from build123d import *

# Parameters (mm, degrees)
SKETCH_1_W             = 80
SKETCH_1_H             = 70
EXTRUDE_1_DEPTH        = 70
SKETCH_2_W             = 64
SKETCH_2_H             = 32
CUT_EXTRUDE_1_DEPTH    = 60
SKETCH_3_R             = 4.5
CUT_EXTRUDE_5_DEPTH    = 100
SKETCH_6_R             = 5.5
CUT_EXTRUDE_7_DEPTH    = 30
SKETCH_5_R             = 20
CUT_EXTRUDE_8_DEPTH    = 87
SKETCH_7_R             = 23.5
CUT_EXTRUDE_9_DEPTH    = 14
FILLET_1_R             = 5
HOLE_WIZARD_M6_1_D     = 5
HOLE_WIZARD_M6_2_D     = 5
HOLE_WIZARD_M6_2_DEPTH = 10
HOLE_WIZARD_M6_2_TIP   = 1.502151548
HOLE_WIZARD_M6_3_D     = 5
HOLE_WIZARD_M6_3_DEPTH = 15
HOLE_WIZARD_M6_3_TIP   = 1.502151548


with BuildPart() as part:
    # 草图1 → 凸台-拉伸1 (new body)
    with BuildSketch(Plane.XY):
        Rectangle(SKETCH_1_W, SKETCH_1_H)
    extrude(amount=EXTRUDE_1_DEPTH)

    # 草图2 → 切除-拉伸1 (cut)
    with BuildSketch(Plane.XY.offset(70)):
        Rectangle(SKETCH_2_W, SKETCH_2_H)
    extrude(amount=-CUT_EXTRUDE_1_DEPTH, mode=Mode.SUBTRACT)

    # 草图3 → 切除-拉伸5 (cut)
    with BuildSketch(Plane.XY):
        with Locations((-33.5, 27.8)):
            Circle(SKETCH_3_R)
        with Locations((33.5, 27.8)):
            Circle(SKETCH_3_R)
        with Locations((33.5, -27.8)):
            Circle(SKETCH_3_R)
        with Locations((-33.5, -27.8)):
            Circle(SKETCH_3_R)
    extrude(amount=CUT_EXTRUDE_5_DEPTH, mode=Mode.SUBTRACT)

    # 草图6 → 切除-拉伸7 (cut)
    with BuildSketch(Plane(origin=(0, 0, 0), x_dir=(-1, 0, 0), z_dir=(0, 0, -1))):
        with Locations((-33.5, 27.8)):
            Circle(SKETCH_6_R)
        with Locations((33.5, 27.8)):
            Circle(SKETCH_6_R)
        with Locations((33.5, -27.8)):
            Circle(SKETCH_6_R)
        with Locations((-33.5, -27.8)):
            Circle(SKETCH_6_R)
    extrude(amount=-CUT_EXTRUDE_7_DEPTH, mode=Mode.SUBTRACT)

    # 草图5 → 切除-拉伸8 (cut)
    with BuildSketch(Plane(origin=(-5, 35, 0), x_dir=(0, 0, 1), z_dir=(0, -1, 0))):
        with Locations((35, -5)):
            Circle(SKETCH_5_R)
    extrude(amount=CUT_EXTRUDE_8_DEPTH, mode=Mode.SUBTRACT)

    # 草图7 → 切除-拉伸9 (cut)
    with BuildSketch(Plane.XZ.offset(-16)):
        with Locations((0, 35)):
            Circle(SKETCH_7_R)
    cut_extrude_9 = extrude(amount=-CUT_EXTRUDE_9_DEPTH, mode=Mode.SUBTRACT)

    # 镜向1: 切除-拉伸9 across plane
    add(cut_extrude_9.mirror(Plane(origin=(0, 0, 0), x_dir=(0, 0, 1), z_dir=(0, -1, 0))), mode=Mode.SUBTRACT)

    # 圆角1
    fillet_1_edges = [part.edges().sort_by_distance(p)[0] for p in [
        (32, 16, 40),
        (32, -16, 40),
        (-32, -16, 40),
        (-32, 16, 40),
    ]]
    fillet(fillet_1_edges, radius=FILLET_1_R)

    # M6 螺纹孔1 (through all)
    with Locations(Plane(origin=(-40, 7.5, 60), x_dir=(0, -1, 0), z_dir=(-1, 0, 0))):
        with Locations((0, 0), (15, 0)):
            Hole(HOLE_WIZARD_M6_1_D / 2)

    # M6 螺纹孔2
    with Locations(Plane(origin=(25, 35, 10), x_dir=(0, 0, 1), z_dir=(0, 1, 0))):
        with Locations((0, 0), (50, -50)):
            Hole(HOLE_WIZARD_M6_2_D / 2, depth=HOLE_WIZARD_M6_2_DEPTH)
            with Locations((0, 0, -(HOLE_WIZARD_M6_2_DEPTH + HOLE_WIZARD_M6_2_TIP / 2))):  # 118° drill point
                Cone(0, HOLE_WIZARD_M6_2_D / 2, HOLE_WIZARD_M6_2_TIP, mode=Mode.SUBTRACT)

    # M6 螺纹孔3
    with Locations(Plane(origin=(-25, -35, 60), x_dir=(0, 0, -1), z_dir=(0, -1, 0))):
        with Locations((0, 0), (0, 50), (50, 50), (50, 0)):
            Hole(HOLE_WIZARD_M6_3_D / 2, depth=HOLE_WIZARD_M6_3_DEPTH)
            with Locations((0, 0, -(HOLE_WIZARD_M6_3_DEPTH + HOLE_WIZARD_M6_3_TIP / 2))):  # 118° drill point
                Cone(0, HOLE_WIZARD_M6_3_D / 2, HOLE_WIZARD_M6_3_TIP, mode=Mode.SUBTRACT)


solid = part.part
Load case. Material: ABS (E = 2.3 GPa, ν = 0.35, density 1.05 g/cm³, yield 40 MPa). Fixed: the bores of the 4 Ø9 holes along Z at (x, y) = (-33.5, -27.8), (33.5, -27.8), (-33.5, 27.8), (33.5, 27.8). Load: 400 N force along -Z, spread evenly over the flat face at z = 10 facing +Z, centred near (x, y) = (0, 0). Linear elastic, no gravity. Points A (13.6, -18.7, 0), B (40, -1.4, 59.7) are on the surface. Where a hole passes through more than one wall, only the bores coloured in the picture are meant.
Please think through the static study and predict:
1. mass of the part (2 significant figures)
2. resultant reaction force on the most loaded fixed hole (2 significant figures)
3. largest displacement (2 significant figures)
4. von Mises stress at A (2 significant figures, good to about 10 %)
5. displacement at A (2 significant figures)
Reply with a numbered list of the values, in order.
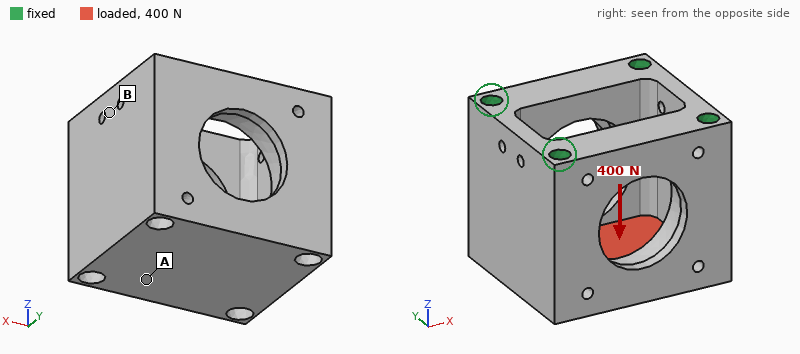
1. 190 g
2. 120 N
3. 26 µm
4. 0.34 MPa
5. 12 µm
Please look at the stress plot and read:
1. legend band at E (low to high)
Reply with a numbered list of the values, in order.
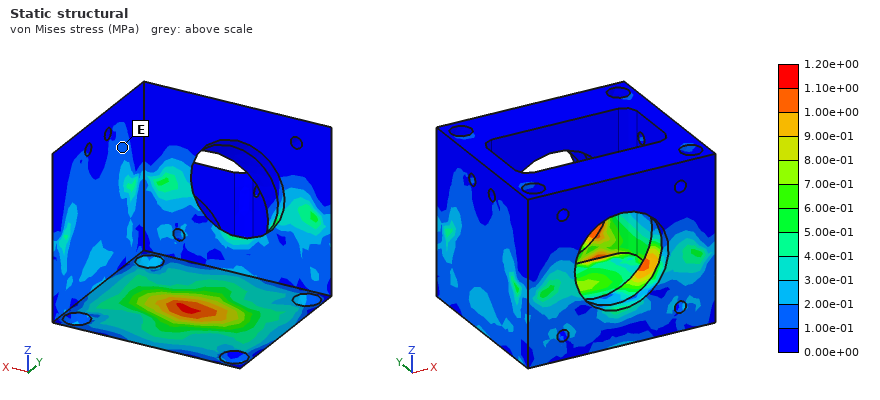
1. 1.00e-01 to 2.00e-01 MPa
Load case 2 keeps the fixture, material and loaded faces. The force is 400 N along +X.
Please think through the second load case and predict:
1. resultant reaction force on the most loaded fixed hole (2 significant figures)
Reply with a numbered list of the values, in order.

1. 110 N
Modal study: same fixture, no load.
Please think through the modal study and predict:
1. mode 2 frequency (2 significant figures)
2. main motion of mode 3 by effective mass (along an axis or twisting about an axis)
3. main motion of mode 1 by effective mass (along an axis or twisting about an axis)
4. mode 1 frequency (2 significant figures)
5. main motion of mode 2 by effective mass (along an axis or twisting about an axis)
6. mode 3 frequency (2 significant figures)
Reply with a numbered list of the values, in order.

1. 2900 Hz
2. twisting about Z
3. along X
4. 2500 Hz
5. along Y
6. 4000 Hz
